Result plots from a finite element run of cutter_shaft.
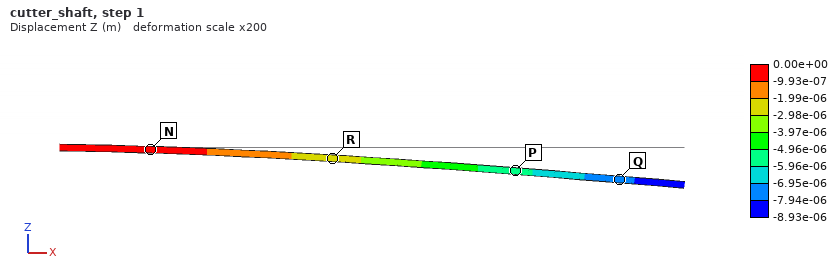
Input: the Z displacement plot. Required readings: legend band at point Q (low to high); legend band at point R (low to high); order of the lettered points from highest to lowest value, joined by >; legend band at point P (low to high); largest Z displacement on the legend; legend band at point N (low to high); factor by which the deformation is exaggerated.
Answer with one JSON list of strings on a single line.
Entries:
["-7.94e-06 to -6.95e-06 m", "-2.98e-06 to -1.99e-06 m", "N > R > P > Q", "-5.96e-06 to -4.96e-06 m", "0.00e+00 m", "-9.93e-07 to 0.00e+00 m", "200"]
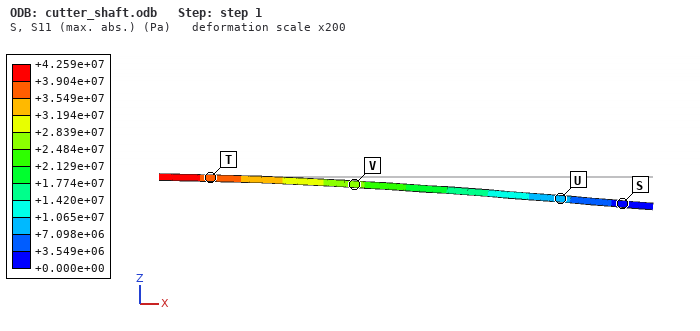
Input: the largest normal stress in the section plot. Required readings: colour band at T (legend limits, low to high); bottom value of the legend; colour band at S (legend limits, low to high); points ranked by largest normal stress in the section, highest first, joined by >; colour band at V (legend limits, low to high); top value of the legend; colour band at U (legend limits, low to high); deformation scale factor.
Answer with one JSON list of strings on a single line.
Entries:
["+3.549e+07 to +3.904e+07 Pa", "+0.000e+00 Pa", "+0.000e+00 to +3.549e+06 Pa", "T > V > U > S", "+2.484e+07 to +2.839e+07 Pa", "+4.259e+07 Pa", "+7.098e+06 to +1.065e+07 Pa", "200"]
